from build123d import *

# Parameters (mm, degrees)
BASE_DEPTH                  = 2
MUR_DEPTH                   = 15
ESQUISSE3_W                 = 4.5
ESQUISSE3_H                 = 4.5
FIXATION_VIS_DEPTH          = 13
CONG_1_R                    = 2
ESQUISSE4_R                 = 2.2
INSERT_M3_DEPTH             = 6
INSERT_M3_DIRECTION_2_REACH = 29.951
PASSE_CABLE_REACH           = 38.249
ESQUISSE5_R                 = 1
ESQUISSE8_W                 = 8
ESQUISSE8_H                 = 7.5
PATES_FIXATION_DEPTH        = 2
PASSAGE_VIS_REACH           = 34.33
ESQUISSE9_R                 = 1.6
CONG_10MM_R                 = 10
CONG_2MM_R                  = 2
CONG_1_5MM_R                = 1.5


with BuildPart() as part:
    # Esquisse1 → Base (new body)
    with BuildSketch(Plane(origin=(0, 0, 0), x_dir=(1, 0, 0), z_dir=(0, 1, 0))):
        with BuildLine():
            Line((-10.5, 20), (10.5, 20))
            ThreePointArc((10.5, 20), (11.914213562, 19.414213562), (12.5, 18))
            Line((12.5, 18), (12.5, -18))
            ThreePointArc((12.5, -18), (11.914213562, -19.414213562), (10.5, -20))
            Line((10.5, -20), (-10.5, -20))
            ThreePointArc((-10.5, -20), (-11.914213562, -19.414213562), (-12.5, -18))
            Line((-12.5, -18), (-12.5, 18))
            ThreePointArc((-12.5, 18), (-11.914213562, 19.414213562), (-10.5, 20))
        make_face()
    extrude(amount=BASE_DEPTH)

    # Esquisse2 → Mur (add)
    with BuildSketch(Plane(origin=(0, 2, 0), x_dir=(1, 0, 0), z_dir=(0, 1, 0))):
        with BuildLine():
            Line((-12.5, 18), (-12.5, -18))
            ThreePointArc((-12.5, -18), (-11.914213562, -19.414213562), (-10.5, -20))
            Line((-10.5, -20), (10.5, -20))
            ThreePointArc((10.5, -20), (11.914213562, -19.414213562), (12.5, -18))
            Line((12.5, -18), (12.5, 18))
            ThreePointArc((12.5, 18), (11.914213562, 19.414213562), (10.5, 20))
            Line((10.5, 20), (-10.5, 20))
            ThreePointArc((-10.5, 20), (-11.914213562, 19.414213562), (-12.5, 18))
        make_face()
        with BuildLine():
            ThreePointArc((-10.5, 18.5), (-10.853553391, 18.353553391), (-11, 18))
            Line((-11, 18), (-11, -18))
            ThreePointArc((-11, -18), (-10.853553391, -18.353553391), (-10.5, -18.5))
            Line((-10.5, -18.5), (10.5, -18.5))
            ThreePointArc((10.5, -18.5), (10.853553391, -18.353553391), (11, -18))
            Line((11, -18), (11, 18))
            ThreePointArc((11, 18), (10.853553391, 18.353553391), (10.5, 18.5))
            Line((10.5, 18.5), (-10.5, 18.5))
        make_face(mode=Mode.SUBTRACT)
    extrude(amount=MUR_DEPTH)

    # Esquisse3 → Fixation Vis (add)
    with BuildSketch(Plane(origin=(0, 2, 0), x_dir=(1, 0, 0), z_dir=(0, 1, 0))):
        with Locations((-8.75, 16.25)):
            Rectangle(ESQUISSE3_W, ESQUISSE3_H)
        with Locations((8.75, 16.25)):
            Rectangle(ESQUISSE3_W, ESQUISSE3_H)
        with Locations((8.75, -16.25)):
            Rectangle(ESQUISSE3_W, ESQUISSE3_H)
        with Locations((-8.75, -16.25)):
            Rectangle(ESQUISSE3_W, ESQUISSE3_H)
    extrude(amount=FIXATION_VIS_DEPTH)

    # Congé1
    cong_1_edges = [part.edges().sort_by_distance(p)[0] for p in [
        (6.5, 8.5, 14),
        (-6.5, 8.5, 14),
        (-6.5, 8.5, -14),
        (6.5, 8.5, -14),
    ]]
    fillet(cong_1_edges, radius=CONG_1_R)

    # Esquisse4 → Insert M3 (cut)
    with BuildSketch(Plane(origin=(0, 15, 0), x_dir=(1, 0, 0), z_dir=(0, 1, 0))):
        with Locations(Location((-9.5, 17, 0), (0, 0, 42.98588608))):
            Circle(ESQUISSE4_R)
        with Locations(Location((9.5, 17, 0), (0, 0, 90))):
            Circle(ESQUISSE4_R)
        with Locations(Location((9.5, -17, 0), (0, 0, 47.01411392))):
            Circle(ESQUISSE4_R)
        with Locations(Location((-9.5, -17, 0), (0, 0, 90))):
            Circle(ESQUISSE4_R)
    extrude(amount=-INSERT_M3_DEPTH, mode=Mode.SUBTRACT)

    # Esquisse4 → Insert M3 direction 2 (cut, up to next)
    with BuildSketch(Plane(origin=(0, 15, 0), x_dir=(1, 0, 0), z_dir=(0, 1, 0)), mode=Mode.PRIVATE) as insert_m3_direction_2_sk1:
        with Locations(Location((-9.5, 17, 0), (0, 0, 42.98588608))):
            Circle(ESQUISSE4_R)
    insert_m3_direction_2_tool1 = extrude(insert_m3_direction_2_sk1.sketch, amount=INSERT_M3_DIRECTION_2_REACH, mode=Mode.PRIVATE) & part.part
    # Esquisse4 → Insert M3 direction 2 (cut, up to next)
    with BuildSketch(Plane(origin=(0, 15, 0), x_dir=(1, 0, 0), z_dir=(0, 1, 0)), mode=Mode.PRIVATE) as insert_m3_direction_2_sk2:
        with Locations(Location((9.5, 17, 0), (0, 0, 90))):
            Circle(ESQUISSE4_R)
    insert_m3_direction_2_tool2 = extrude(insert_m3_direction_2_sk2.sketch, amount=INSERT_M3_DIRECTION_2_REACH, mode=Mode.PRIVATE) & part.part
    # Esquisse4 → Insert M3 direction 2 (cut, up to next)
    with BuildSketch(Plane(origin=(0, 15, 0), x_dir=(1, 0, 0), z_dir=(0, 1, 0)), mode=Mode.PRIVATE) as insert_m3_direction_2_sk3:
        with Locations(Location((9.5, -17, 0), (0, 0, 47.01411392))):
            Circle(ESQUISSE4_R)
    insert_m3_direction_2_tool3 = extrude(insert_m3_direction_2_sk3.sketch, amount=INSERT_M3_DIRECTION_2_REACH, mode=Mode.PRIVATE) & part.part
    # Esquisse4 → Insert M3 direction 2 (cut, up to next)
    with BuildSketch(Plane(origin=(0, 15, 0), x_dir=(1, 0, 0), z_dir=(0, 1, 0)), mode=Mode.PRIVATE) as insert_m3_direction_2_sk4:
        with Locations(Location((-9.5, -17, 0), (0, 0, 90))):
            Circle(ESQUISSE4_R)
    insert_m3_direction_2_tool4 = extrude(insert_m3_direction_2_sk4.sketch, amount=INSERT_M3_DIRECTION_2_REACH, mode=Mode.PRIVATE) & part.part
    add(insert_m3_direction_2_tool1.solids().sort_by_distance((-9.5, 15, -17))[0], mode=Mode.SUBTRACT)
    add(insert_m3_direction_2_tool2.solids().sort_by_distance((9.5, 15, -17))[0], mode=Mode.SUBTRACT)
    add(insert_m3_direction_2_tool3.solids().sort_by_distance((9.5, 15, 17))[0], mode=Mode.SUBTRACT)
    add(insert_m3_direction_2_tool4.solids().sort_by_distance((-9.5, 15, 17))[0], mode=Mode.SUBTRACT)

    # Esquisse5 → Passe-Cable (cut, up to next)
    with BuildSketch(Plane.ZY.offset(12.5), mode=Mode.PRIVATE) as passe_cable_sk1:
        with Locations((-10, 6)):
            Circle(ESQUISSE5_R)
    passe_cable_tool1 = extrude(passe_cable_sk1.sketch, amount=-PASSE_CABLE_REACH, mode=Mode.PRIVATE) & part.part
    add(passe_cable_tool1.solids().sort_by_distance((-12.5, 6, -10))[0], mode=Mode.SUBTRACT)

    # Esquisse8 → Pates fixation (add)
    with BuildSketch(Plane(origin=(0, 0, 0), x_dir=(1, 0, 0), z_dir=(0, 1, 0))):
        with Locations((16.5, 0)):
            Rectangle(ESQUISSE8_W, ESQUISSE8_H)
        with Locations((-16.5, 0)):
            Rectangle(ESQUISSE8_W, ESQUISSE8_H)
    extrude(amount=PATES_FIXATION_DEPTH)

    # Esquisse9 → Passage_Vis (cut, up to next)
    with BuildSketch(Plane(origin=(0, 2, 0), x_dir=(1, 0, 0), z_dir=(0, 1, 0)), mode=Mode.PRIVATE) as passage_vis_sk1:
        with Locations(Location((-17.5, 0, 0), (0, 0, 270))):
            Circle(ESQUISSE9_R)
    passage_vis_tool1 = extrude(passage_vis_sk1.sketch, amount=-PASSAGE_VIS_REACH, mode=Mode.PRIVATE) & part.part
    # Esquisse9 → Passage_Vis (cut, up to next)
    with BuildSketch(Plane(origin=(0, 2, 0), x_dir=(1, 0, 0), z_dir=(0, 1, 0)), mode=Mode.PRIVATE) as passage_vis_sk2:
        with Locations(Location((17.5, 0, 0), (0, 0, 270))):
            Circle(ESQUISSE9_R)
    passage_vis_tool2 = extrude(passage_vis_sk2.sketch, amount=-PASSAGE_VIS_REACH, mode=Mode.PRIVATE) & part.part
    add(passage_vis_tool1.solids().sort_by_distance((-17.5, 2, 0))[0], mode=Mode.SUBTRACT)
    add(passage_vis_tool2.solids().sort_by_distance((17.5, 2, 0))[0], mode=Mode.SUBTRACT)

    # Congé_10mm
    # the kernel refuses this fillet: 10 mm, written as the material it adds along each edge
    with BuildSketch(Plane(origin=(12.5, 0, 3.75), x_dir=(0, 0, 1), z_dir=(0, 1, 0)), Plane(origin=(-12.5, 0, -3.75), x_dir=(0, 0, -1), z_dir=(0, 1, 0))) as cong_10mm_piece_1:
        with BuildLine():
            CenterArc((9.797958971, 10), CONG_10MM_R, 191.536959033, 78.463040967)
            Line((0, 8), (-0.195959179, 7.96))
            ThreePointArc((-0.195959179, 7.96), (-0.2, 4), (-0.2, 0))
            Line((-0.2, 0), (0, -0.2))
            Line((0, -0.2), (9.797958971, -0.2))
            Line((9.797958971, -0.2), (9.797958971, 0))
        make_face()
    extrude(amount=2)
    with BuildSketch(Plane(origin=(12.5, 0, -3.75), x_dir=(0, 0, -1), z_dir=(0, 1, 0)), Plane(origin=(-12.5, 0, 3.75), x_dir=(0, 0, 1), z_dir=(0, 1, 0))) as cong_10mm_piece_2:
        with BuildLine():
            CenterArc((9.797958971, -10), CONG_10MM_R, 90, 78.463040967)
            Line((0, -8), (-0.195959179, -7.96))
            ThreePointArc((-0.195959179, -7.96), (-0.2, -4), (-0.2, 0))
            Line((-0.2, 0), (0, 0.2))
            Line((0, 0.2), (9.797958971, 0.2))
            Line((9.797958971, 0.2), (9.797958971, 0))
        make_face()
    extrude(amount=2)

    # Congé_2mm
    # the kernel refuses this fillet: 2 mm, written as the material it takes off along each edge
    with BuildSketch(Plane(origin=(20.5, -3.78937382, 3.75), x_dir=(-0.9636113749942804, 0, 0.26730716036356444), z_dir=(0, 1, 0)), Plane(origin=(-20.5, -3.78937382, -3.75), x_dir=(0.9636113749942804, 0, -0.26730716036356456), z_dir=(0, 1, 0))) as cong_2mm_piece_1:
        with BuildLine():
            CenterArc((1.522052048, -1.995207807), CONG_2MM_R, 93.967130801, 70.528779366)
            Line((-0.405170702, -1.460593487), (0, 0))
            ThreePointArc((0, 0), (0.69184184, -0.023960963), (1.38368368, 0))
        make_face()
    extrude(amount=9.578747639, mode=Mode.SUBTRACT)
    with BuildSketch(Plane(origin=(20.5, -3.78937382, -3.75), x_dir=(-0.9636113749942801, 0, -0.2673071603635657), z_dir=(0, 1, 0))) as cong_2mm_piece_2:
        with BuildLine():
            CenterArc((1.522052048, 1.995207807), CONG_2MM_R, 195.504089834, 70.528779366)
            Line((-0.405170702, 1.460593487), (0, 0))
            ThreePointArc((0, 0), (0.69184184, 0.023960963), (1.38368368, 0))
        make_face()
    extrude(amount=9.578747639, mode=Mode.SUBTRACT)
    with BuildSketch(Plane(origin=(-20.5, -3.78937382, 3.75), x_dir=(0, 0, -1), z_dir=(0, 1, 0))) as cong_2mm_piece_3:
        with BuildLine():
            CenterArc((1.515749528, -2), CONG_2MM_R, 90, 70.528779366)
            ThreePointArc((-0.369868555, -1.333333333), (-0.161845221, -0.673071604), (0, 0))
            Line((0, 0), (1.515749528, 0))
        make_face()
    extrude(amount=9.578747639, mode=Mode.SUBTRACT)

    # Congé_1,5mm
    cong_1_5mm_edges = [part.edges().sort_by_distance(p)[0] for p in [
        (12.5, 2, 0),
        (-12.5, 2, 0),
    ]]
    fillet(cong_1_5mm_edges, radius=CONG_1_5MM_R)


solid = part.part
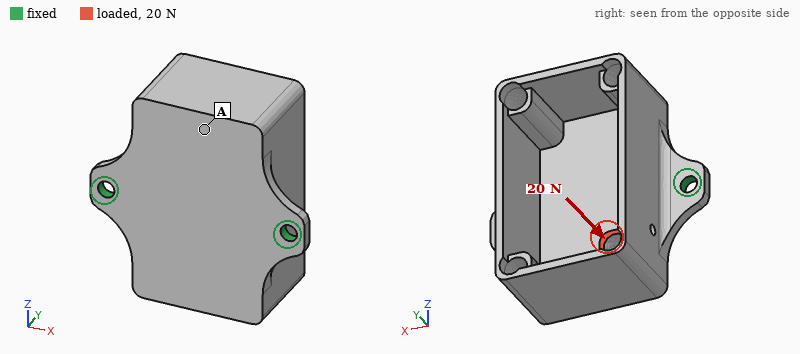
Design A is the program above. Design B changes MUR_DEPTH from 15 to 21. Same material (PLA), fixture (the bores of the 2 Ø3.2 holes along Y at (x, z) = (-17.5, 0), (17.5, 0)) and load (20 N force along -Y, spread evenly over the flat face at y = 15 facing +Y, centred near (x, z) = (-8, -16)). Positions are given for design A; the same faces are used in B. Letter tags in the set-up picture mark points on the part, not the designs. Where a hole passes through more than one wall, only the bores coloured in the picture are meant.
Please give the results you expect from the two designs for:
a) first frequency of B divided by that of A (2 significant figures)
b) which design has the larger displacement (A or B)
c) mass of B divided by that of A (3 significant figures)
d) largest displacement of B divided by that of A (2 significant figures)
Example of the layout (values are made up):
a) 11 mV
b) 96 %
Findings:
a) 0.83
b) B
c) 1.18
d) 1.1
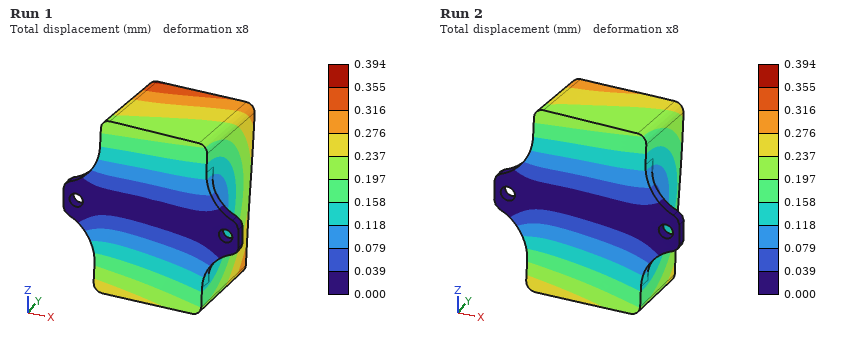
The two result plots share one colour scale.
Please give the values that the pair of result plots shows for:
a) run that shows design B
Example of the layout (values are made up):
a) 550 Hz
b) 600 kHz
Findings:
a) Run 1
